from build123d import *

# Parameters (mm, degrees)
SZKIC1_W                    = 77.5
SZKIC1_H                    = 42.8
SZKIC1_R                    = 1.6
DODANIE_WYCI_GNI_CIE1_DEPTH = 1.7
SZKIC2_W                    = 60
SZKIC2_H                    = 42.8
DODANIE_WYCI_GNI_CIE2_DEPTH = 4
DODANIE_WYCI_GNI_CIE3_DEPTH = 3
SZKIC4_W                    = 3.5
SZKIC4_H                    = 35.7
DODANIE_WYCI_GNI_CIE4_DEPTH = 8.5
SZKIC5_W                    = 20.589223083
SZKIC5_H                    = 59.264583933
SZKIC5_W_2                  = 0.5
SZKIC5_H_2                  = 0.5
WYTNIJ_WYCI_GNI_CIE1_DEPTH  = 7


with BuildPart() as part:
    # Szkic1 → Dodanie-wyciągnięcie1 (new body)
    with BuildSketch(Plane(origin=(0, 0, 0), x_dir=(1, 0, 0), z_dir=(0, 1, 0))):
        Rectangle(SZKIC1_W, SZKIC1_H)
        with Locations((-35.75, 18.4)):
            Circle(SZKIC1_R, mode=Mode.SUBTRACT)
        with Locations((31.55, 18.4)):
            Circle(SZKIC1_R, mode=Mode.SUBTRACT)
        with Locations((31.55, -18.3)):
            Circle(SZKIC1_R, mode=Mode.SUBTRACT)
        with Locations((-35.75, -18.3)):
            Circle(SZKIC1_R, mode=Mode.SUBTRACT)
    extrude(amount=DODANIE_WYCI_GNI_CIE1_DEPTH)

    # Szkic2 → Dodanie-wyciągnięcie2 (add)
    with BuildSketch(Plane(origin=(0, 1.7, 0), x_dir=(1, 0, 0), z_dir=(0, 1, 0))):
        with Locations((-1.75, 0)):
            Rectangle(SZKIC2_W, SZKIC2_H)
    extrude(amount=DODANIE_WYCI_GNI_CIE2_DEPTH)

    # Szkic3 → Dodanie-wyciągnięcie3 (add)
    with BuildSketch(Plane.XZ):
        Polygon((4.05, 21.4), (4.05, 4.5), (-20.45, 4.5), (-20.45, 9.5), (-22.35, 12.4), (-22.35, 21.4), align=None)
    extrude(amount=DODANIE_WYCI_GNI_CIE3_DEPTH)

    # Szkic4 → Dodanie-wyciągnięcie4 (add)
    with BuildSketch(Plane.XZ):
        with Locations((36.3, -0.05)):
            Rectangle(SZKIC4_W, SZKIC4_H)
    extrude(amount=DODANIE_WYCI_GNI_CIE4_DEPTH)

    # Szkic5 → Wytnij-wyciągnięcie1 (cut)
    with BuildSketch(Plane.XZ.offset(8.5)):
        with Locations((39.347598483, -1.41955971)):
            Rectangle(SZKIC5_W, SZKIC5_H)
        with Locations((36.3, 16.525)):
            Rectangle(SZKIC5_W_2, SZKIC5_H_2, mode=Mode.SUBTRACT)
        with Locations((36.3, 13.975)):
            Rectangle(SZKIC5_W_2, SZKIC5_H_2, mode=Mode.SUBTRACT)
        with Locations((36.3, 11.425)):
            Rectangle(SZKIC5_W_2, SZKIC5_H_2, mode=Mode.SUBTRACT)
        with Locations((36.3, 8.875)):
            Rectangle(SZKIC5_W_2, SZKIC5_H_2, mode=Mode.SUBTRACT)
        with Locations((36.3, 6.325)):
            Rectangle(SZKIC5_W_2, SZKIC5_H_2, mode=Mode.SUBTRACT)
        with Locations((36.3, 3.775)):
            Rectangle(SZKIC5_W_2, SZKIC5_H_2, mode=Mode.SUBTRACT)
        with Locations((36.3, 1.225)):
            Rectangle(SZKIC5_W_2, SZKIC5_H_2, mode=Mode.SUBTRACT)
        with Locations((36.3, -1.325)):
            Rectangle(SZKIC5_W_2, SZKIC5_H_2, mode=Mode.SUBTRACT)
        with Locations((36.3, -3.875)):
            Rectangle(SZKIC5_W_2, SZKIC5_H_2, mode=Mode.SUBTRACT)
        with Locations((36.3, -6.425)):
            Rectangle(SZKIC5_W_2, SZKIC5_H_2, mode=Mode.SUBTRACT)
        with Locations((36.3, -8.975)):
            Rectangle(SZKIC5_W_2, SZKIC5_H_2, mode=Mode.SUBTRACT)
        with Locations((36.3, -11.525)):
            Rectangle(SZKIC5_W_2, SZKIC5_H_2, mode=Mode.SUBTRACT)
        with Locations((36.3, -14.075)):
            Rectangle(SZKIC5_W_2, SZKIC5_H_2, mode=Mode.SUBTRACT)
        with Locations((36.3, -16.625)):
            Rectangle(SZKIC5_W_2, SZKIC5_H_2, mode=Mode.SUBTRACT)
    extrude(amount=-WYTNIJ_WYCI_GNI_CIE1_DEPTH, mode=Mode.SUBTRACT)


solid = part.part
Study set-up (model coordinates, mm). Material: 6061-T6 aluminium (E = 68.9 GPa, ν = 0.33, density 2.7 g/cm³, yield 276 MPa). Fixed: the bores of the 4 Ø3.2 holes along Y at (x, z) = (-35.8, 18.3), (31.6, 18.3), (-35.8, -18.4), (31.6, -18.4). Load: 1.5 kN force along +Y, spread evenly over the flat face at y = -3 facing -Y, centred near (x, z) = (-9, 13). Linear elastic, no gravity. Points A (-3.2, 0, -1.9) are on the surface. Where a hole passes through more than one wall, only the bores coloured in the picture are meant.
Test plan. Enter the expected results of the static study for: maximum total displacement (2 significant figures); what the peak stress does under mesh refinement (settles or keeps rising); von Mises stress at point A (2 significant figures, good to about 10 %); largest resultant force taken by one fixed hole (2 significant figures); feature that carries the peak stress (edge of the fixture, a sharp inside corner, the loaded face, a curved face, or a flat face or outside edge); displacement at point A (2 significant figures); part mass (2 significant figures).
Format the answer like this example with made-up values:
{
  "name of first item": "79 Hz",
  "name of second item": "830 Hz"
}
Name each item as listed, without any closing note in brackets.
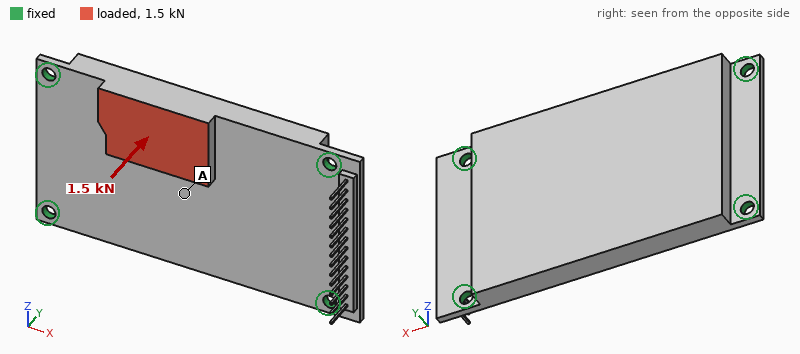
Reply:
{
  "maximum total displacement": "0.13 mm",
  "what the peak stress does under mesh refinement": "keeps rising",
  "von Mises stress at point A": "23 MPa",
  "largest resultant force taken by one fixed hole": "1.1 kN",
  "feature that carries the peak stress": "edge of the fixture",
  "displacement at point A": "0.077 mm",
  "part mass": "47 g"
}
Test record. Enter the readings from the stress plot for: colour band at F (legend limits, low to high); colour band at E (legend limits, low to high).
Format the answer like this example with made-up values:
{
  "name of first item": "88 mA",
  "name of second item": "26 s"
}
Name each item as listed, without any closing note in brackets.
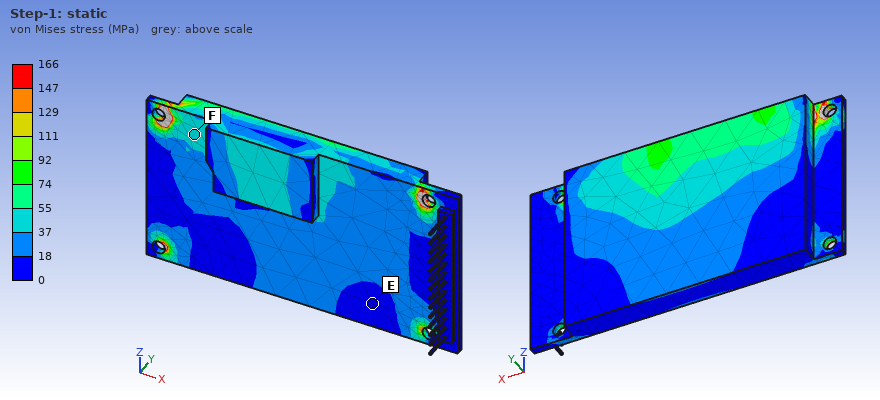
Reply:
{
  "colour band at F": "37 to 55 MPa",
  "colour band at E": "0 to 18 MPa"
}
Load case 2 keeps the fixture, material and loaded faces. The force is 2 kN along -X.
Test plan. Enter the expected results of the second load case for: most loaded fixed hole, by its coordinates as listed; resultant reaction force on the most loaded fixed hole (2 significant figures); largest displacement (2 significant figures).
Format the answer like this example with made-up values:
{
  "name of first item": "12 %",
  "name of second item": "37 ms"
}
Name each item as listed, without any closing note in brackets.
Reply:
{
  "most loaded fixed hole, by its coordinates as listed": "(-35.8, 18.3)",
  "resultant reaction force on the most loaded fixed hole": "770 N",
  "largest displacement": "30 µm"
}
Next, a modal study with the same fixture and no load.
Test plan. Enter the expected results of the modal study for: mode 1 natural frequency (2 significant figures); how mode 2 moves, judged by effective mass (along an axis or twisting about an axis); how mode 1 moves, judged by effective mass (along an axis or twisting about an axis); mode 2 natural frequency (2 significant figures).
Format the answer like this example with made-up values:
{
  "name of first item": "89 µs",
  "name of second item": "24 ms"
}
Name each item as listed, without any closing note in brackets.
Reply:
{
  "mode 1 natural frequency": "3900 Hz",
  "how mode 2 moves, judged by effective mass": "twisting about X",
  "how mode 1 moves, judged by effective mass": "along Y",
  "mode 2 natural frequency": "6400 Hz"
}
